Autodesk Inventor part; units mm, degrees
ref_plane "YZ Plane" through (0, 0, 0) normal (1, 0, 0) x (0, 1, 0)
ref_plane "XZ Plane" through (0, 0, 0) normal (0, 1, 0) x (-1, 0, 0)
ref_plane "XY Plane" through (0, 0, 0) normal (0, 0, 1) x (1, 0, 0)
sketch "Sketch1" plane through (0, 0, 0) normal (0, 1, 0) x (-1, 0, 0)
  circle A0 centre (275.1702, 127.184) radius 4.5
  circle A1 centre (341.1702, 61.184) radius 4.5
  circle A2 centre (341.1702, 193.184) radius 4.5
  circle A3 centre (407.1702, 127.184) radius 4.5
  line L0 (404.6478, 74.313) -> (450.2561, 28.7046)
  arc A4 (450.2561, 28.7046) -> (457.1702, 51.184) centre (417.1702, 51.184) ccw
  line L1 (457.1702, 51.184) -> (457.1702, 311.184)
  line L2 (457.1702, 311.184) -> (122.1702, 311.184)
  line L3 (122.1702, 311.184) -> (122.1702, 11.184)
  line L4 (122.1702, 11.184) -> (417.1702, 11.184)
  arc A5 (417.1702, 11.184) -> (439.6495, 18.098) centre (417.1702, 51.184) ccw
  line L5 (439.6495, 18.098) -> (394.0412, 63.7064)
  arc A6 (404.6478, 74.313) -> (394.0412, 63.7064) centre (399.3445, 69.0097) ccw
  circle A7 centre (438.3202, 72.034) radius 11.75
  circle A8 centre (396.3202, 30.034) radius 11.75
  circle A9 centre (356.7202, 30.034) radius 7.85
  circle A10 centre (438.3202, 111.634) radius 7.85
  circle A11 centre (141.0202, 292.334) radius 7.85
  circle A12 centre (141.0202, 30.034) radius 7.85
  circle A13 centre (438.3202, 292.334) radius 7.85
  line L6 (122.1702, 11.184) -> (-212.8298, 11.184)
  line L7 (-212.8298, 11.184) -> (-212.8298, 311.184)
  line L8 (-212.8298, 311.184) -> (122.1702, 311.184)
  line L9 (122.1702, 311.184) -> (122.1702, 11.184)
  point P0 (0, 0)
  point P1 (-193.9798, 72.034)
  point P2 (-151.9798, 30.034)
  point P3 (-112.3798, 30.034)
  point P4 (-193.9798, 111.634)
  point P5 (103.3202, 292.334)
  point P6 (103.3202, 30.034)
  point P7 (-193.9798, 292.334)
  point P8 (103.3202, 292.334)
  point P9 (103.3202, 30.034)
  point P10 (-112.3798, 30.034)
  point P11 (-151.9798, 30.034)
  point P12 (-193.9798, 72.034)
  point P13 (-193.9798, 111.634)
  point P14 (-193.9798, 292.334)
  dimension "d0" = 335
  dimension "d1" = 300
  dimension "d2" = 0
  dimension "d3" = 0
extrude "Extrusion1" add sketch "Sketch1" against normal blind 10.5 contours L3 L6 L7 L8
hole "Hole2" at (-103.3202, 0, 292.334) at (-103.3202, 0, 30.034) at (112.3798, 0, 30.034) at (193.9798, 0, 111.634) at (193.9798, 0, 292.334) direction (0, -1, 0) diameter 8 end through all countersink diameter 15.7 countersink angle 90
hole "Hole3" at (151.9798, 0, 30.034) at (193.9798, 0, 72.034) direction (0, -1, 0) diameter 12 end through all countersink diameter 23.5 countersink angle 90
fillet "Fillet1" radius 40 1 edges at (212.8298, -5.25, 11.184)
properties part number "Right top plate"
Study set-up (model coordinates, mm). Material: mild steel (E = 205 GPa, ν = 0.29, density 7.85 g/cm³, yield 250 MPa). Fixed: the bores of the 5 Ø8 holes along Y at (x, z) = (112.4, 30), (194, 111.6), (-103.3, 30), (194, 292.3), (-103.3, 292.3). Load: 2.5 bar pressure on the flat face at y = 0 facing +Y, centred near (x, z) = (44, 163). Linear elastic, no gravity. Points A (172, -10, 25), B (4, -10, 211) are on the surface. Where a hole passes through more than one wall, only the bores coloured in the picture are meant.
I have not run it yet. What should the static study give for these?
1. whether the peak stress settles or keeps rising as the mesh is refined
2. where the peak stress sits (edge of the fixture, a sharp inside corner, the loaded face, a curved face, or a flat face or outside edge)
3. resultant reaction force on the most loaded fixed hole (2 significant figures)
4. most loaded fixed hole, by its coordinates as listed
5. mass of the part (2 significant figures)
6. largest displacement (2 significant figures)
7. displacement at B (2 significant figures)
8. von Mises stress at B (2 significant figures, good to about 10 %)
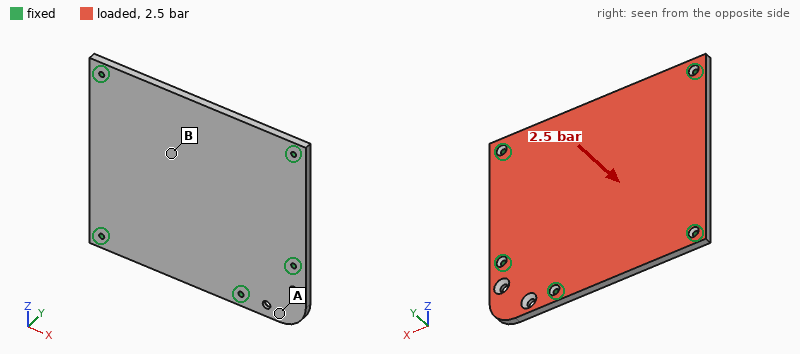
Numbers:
keeps rising
edge of the fixture
8.5 kN
(-103.3, 292.3)
8.2 kg
0.52 mm
0.51 mm
56 MPa
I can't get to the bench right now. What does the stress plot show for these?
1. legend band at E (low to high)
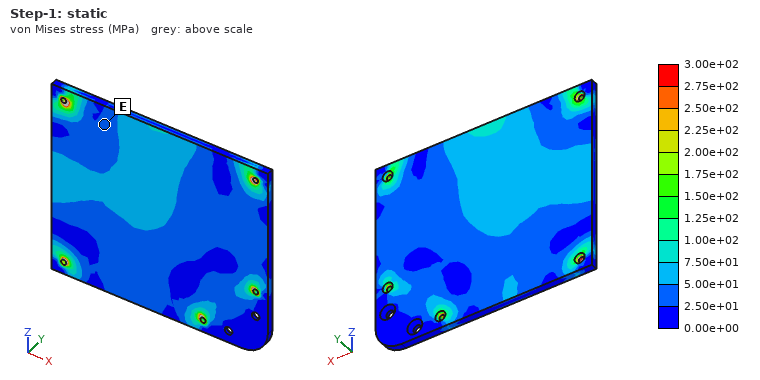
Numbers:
2.50e+01 to 5.00e+01 MPa
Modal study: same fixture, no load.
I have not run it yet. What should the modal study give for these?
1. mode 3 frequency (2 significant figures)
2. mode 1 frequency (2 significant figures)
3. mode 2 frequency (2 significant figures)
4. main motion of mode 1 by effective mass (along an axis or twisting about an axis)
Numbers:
970 Hz
450 Hz
720 Hz
along Y
